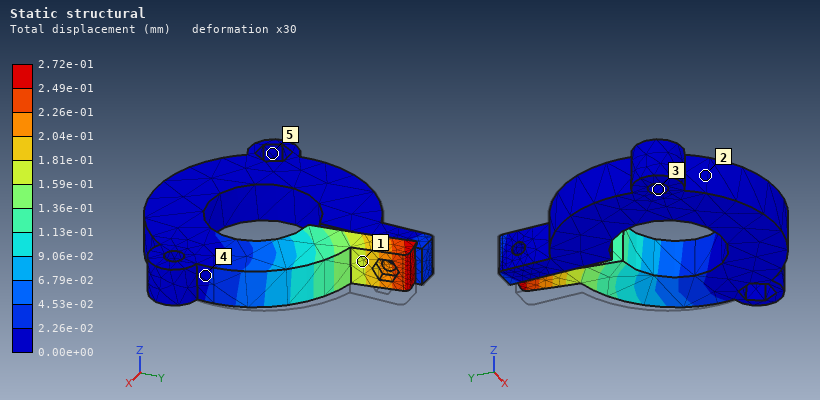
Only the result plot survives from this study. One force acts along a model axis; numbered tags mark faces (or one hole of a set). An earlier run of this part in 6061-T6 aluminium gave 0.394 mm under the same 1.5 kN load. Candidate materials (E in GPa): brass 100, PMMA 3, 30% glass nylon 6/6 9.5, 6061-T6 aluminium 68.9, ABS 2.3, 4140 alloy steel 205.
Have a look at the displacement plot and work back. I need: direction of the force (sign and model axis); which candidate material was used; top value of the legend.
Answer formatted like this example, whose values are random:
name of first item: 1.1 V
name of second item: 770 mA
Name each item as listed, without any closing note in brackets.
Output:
direction of the force: -X
which candidate material was used: brass
top value of the legend: 2.72e-01 mm
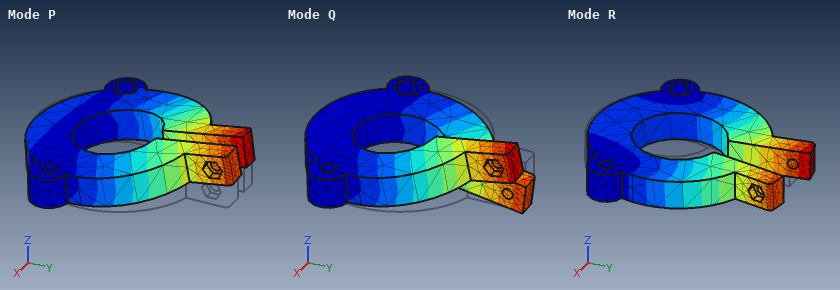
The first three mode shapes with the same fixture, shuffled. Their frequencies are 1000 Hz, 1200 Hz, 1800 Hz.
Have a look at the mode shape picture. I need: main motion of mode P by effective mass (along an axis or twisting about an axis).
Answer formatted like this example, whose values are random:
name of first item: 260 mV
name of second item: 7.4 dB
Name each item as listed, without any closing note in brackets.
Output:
main motion of mode P by effective mass: along Z
